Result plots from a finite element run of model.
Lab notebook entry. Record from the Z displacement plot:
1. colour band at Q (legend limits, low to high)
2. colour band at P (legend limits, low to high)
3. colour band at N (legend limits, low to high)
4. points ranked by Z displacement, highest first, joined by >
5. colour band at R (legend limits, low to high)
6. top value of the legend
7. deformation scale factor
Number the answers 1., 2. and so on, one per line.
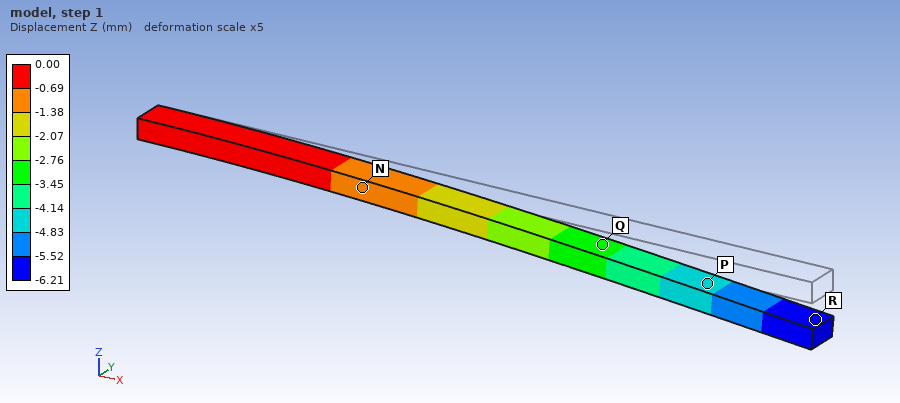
1. -3.45 to -2.76 mm
2. -4.83 to -4.14 mm
3. -1.38 to -0.69 mm
4. N > Q > P > R
5. -6.21 to -5.52 mm
6. 0.00 mm
7. 5
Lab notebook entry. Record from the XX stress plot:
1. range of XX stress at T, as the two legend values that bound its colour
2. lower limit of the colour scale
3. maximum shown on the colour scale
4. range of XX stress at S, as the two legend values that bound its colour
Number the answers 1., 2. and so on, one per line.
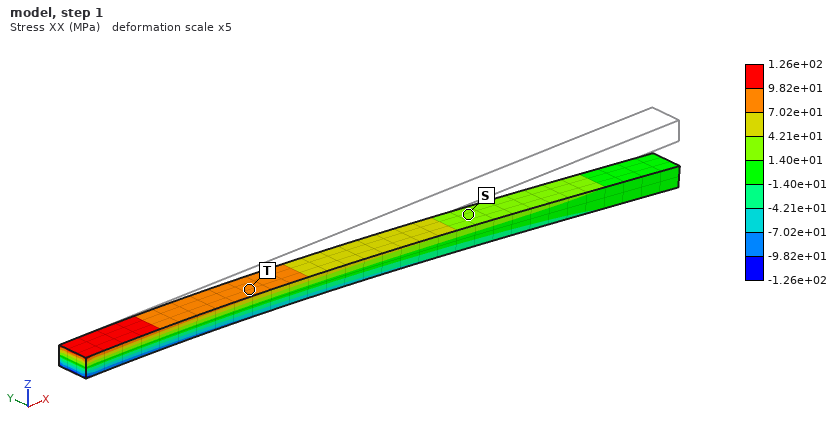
1. 7.02e+01 to 9.82e+01 MPa
2. -1.26e+02 MPa
3. 1.26e+02 MPa
4. 1.40e+01 to 4.21e+01 MPa
